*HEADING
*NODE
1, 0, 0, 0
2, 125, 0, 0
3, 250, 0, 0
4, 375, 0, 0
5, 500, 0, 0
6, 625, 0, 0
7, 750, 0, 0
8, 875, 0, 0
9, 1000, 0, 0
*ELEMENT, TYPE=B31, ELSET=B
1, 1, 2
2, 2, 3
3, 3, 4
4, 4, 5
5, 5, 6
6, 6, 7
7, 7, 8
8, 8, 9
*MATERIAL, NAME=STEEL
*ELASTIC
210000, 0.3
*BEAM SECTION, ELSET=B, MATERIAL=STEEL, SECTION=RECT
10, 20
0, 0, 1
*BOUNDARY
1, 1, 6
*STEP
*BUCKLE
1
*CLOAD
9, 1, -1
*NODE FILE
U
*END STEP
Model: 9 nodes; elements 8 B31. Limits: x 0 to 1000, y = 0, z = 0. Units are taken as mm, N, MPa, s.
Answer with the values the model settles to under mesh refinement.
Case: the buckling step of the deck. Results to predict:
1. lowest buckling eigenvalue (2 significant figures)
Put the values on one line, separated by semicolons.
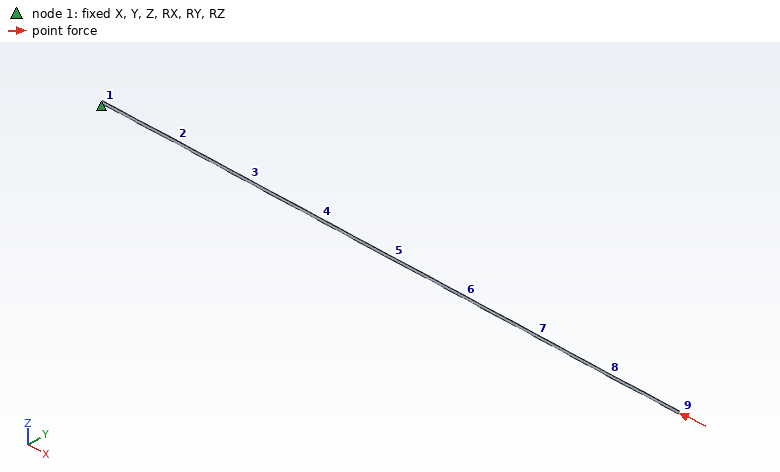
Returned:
860
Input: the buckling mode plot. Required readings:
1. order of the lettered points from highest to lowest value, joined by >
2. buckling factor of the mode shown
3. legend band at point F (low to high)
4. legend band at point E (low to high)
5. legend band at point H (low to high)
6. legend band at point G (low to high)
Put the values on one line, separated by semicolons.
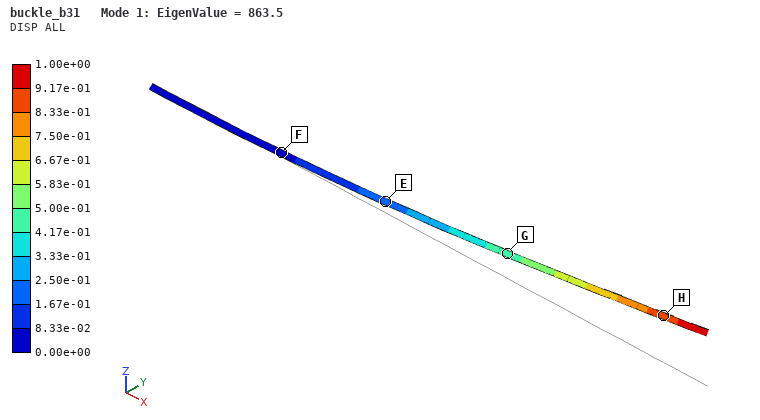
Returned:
H > G > E > F; 863.5; 0.00e+00 to 8.33e-02; 1.67e-01 to 2.50e-01; 8.33e-01 to 9.17e-01; 4.17e-01 to 5.00e-01
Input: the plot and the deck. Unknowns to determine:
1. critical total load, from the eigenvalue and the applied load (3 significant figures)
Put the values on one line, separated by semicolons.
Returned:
864 N
